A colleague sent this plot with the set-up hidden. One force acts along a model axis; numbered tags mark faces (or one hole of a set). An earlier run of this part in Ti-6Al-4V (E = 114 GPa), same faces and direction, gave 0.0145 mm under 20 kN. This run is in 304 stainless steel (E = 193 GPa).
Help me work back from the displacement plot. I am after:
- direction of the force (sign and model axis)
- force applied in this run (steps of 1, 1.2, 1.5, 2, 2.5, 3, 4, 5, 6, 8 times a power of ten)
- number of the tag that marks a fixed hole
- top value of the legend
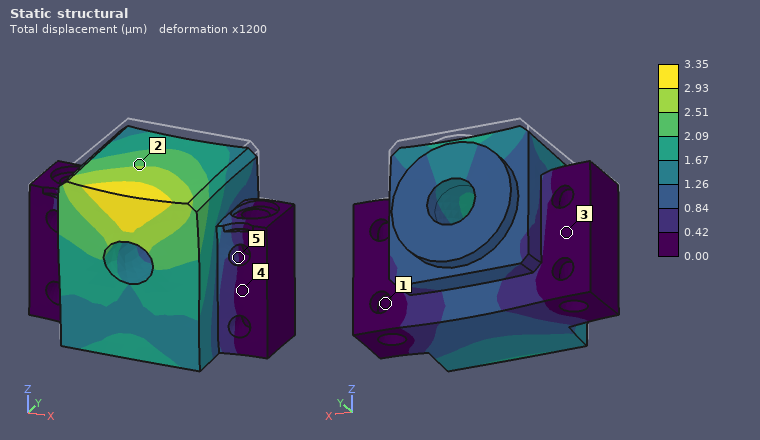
-Z
8 kN
1
3.35 µm
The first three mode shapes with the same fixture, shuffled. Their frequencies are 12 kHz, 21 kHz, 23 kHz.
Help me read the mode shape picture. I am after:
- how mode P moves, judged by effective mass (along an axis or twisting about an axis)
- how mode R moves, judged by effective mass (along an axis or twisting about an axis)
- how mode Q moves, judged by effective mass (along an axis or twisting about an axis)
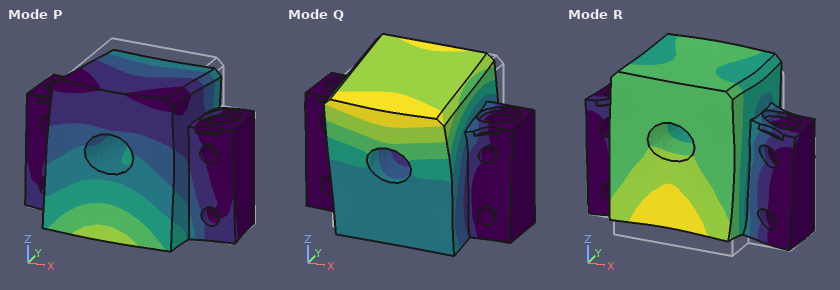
along Y
along Z
along Y
